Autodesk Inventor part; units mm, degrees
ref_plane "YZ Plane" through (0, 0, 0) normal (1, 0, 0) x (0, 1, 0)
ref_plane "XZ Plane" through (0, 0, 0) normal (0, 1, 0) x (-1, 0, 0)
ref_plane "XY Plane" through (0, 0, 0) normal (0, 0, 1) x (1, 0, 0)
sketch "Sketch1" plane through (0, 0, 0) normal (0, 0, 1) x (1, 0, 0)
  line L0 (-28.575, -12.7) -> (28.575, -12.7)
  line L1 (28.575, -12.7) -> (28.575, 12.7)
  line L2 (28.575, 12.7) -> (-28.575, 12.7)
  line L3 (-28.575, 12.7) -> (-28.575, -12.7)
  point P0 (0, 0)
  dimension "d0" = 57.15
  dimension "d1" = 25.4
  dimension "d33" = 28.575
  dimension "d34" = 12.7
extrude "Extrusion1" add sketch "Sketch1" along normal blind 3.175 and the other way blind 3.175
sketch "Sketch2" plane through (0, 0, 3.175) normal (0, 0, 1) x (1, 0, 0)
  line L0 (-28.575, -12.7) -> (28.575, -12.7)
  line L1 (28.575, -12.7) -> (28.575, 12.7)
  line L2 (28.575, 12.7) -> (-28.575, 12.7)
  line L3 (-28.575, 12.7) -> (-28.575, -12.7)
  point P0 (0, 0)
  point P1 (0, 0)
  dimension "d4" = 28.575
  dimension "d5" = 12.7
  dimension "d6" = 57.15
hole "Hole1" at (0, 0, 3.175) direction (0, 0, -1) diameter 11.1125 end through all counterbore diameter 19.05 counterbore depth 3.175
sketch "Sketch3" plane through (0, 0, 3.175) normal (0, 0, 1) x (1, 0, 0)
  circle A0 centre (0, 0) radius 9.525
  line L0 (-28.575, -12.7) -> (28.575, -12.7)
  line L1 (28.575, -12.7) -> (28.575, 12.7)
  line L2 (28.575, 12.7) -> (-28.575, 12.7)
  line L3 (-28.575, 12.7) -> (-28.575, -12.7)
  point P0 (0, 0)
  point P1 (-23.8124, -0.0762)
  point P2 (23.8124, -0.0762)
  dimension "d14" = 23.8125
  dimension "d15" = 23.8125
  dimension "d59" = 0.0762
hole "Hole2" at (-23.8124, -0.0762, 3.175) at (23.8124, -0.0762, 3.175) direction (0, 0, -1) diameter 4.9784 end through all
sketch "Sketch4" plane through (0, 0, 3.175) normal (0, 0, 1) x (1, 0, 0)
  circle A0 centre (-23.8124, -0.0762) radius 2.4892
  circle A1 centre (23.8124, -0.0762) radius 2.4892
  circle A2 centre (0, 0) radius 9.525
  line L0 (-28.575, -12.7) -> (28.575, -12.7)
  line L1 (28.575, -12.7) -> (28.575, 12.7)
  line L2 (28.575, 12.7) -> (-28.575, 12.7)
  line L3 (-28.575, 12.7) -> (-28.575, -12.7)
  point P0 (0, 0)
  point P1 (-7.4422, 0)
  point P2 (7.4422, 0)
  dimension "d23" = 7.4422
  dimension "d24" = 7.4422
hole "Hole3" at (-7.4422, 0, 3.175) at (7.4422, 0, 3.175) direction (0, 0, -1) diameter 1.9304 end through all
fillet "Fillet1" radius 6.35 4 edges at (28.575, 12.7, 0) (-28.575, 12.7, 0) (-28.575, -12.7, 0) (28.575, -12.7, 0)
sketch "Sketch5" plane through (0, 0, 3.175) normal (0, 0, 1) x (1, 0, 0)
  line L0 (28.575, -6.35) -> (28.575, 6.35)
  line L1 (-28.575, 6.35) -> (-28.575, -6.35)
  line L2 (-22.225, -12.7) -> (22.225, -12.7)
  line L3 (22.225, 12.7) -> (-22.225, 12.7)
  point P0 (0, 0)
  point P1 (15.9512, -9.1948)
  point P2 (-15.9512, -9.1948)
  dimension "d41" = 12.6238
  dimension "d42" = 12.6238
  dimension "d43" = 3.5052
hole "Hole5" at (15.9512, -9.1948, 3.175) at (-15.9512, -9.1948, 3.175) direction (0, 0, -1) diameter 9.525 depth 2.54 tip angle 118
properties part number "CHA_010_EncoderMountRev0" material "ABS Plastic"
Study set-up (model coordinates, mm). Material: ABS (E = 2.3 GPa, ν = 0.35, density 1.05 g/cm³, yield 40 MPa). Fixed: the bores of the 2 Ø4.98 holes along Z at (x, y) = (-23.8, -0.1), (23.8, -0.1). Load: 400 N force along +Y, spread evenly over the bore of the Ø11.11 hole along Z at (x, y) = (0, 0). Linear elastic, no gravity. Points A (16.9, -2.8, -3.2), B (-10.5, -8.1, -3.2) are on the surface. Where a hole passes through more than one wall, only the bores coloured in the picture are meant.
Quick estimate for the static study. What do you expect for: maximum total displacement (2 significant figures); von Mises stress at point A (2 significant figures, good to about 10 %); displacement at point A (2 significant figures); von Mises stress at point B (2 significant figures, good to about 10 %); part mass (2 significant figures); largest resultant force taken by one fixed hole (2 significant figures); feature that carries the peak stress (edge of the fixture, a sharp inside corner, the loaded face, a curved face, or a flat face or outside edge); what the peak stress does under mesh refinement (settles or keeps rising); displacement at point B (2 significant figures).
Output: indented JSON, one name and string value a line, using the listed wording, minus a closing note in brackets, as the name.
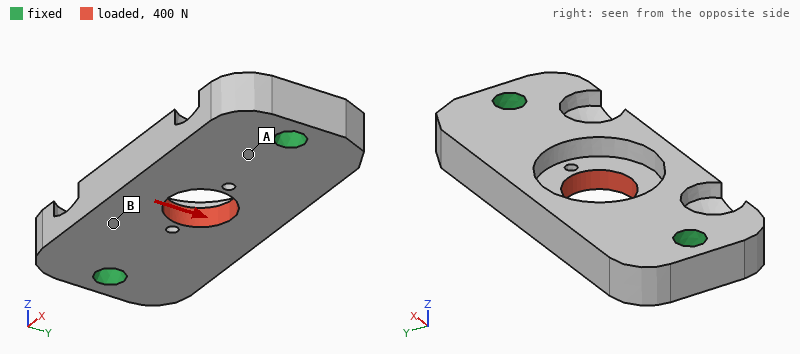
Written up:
{
  "maximum total displacement": "0.10 mm",
  "von Mises stress at point A": "5.4 MPa",
  "displacement at point A": "0.030 mm",
  "von Mises stress at point B": "3.5 MPa",
  "part mass": "7.4 g",
  "largest resultant force taken by one fixed hole": "200 N",
  "feature that carries the peak stress": "edge of the fixture",
  "what the peak stress does under mesh refinement": "keeps rising",
  "displacement at point B": "0.064 mm"
}
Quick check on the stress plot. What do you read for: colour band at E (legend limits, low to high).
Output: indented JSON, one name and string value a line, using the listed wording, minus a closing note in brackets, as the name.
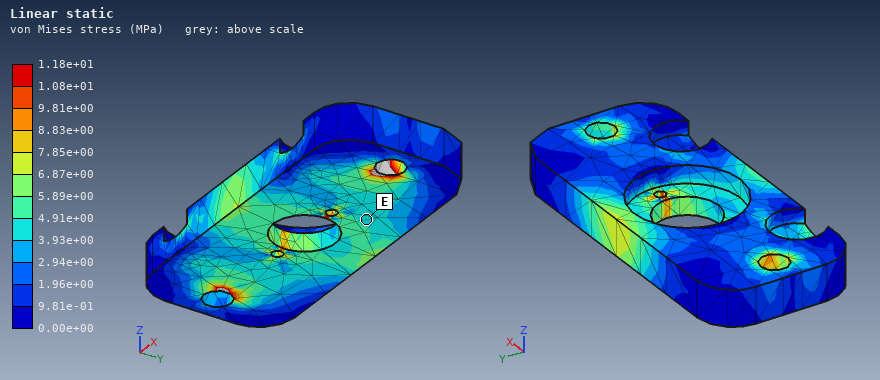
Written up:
{
  "colour band at E": "3.93e+00 to 4.91e+00 MPa"
}
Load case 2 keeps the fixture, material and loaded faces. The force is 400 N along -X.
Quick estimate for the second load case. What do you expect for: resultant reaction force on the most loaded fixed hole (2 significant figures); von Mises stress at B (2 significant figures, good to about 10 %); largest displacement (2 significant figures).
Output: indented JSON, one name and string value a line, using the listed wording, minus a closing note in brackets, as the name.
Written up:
{
  "resultant reaction force on the most loaded fixed hole": "200 N",
  "von Mises stress at B": "2.2 MPa",
  "largest displacement": "32 µm"
}
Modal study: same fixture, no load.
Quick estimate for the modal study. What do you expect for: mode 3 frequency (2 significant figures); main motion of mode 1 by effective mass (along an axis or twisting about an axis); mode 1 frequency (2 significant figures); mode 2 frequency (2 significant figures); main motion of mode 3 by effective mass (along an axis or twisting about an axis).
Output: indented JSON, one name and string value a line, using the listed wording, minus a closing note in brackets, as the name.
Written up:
{
  "mode 3 frequency": "7000 Hz",
  "main motion of mode 1 by effective mass": "along Z",
  "mode 1 frequency": "3700 Hz",
  "mode 2 frequency": "4000 Hz",
  "main motion of mode 3 by effective mass": "along Y"
}
